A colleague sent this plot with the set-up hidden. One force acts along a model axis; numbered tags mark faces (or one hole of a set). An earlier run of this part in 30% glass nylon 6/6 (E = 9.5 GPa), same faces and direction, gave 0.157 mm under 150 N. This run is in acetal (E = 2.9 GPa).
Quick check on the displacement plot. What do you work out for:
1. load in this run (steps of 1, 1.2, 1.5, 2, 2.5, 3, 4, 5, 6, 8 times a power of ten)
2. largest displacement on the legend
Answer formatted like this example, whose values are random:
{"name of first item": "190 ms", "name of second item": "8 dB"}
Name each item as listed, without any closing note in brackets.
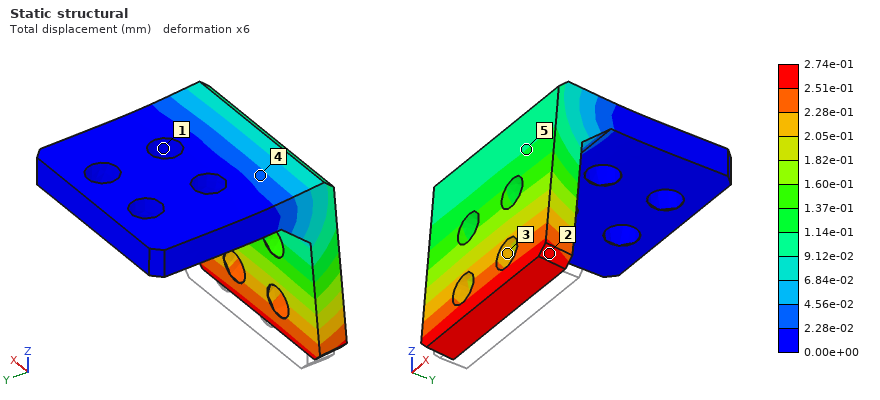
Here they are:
{"load in this run": "80 N", "largest displacement on the legend": "2.74e-01 mm"}
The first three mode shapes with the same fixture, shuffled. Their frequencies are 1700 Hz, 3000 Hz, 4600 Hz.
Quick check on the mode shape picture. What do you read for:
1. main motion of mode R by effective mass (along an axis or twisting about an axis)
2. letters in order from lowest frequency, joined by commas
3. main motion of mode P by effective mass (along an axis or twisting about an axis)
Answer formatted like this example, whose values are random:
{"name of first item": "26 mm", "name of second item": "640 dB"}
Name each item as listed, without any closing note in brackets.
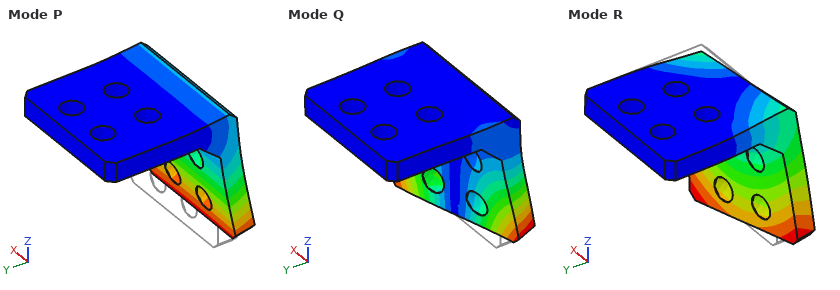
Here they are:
{"main motion of mode R by effective mass": "along X", "letters in order from lowest frequency, joined by commas": "P, R, Q", "main motion of mode P by effective mass": "along Y"}
